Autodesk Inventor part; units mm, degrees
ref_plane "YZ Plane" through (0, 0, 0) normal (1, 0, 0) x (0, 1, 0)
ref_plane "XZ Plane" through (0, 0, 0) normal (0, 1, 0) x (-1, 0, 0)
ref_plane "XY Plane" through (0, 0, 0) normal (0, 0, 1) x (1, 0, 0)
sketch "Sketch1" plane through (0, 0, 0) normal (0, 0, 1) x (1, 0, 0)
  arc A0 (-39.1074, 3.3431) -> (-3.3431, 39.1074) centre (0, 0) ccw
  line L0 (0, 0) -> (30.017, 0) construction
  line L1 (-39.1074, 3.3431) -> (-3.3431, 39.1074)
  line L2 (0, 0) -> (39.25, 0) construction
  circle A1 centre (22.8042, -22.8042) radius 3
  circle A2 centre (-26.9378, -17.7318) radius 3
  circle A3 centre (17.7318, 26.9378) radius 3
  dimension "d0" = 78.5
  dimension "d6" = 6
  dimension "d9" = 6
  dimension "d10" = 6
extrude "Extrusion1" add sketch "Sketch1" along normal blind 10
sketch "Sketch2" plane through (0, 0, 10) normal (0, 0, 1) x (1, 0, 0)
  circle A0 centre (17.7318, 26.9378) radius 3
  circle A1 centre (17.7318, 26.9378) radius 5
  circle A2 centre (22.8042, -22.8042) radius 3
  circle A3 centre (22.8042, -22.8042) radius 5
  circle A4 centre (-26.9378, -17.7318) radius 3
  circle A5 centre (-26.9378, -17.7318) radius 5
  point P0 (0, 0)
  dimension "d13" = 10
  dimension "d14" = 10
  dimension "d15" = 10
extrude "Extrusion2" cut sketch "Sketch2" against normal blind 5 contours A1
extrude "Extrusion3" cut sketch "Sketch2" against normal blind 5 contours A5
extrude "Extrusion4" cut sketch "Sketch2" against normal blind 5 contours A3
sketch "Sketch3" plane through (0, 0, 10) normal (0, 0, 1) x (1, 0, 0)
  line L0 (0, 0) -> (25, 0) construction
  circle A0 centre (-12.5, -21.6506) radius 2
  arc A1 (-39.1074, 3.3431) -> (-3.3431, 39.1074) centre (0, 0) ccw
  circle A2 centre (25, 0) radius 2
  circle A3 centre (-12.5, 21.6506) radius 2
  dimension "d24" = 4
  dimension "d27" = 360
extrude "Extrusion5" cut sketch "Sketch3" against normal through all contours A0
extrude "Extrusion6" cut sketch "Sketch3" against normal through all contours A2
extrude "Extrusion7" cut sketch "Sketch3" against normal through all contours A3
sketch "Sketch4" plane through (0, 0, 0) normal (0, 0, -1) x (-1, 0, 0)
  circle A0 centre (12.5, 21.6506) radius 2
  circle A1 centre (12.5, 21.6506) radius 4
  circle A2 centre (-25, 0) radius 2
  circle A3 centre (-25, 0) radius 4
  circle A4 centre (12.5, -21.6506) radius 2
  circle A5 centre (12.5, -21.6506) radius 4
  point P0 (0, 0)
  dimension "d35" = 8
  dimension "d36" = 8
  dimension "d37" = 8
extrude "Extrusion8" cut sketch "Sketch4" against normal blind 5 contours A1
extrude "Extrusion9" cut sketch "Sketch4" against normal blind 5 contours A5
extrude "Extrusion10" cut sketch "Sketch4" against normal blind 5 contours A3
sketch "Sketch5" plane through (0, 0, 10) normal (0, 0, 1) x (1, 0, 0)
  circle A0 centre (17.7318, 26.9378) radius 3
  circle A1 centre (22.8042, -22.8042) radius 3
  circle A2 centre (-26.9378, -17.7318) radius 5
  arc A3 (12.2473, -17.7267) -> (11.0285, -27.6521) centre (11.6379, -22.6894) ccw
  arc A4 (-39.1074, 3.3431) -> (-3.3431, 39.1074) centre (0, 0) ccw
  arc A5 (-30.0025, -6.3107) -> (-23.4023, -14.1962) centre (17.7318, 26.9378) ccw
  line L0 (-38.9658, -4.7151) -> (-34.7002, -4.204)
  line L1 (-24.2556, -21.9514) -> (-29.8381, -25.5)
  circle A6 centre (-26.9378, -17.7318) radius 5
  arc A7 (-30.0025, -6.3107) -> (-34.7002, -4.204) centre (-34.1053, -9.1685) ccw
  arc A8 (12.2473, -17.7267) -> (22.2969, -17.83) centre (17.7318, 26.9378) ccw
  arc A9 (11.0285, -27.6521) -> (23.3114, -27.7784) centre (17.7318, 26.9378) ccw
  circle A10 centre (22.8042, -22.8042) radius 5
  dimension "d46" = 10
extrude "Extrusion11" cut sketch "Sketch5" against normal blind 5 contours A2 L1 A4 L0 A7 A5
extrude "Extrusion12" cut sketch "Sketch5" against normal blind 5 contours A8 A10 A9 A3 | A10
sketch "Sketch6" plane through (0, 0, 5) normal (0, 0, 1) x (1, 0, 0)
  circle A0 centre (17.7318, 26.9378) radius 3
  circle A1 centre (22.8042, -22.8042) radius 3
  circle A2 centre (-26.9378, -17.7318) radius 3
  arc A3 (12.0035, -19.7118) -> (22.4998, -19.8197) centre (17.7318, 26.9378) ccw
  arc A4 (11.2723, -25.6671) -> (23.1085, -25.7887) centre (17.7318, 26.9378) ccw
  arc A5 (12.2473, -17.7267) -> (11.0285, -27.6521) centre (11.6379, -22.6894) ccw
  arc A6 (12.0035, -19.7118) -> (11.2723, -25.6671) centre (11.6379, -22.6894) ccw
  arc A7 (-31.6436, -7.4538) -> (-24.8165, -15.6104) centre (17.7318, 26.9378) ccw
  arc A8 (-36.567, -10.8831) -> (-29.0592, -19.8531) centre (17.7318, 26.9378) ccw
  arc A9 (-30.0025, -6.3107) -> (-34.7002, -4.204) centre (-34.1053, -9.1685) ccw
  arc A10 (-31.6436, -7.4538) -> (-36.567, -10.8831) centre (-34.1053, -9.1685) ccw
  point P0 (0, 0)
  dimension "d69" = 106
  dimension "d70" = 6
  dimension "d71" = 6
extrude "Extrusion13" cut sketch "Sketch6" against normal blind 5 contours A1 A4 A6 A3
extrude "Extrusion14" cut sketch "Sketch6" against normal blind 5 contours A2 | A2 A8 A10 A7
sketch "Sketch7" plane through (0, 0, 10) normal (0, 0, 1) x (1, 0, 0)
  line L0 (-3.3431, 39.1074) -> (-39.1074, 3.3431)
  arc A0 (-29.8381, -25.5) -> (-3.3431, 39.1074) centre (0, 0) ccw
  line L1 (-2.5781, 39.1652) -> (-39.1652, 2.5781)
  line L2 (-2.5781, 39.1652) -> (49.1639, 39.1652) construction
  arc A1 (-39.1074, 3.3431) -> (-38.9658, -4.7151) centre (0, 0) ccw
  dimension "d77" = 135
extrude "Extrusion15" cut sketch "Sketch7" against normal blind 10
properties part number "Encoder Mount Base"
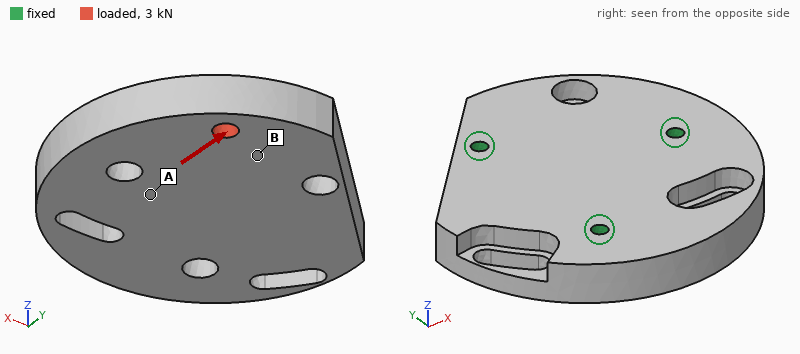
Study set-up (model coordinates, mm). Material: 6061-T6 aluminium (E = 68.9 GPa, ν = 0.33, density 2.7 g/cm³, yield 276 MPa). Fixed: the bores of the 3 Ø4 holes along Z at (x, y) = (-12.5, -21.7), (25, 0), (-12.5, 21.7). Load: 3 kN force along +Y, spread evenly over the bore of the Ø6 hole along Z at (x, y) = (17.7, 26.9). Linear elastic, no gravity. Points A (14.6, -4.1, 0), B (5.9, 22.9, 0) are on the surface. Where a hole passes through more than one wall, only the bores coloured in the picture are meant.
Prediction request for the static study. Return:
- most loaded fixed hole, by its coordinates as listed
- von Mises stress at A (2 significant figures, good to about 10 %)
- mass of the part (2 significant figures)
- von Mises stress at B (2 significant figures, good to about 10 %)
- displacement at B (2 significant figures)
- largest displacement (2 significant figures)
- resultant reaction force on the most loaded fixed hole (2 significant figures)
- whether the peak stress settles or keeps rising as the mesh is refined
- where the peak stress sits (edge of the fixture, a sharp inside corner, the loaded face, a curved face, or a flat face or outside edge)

(25, 0)
7.8 MPa
110 g
16 MPa
9.9 µm
26 µm
1.8 kN
keeps rising
edge of the fixture
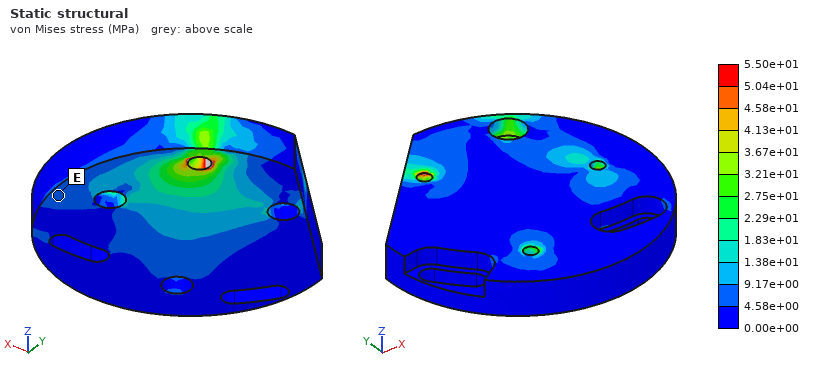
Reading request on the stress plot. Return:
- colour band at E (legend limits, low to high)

4.58e+00 to 9.17e+00 MPa
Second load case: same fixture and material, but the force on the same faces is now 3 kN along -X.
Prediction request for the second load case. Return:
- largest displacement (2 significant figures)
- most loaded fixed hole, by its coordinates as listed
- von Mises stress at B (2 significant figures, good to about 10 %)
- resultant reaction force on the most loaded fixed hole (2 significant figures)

17 µm
(-12.5, 21.7)
20 MPa
2.0 kN
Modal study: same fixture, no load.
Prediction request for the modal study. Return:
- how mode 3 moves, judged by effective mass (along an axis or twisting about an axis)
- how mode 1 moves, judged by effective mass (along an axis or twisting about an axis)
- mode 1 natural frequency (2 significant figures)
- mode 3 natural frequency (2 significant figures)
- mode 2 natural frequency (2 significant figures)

along Z
twisting about X
7000 Hz
11 kHz
7800 Hz
